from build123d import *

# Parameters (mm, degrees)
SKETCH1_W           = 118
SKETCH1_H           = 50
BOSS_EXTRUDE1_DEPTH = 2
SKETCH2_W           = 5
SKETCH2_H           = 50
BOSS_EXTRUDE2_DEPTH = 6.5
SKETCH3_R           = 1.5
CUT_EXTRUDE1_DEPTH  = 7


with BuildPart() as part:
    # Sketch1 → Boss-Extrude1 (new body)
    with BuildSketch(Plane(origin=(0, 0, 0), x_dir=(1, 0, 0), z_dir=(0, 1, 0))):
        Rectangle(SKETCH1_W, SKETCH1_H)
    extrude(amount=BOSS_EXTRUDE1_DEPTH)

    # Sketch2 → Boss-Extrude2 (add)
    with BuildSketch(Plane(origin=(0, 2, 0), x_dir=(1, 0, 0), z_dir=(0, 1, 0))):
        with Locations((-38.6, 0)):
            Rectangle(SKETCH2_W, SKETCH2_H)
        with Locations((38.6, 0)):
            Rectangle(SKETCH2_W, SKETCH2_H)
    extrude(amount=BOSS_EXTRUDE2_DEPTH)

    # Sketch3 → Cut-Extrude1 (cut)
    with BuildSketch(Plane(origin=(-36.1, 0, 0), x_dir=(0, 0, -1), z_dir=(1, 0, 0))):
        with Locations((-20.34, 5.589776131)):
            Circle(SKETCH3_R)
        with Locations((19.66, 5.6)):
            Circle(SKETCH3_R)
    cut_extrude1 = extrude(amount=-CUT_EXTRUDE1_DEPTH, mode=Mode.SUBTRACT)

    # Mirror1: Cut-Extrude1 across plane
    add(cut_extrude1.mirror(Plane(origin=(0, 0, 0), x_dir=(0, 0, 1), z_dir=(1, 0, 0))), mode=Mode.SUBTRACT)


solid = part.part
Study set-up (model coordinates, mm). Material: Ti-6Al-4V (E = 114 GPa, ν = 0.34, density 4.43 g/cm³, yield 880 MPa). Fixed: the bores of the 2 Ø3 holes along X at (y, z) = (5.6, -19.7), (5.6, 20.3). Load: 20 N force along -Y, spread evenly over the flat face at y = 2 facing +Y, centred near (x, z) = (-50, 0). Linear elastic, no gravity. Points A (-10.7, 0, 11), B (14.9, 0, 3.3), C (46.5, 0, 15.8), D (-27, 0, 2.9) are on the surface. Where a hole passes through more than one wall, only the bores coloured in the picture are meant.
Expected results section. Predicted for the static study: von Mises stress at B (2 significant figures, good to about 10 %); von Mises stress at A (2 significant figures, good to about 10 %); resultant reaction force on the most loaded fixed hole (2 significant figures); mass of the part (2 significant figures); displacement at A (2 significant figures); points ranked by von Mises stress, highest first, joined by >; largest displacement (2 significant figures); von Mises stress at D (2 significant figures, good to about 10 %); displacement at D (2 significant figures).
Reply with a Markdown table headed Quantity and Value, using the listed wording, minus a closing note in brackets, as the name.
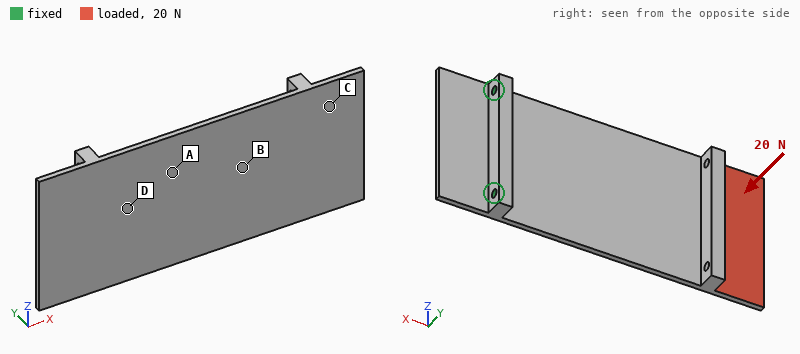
| Quantity | Value |
|---|---|
| von Mises stress at B | 35 MPa |
| von Mises stress at A | 22 MPa |
| resultant reaction force on the most loaded fixed hole | 28 N |
| mass of the part | 66 g |
| displacement at A | 0.42 mm |
| points ranked by von Mises stress, highest first, joined by > | B > A > D > C |
| largest displacement | 1.3 mm |
| von Mises stress at D | 13 MPa |
| displacement at D | 0.69 mm |
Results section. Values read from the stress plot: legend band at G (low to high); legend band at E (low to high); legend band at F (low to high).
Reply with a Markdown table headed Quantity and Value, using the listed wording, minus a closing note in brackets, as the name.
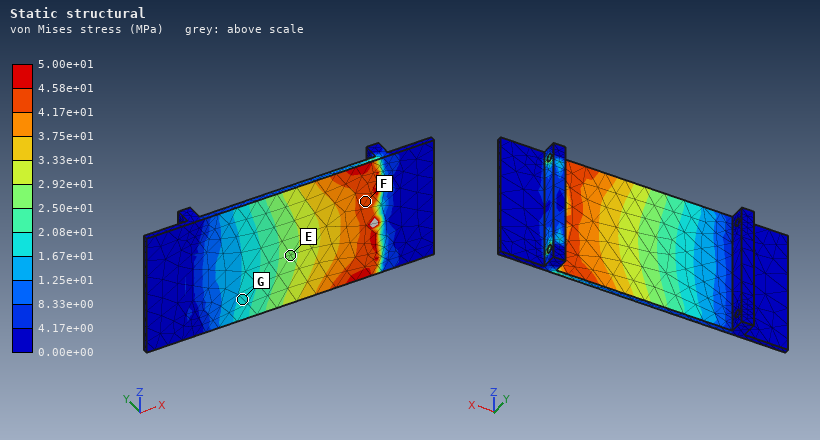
| Quantity | Value |
|---|---|
| legend band at G | 1.67e+01 to 2.08e+01 MPa |
| legend band at E | 2.50e+01 to 2.92e+01 MPa |
| legend band at F | 4.17e+01 to 4.58e+01 MPa |
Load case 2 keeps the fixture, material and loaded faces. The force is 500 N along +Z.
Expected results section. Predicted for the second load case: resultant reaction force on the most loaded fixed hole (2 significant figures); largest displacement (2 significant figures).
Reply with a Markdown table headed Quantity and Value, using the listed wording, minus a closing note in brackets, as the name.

| Quantity | Value |
|---|---|
| resultant reaction force on the most loaded fixed hole | 1.1 kN |
| largest displacement | 0.18 mm |
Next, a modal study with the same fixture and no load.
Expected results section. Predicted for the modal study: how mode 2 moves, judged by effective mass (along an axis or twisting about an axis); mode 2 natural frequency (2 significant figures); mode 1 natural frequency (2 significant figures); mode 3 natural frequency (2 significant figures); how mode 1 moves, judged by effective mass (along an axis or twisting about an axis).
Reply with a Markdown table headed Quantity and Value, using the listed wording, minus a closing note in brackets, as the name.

| Quantity | Value |
|---|---|
| how mode 2 moves, judged by effective mass | twisting about X |
| mode 2 natural frequency | 670 Hz |
| mode 1 natural frequency | 160 Hz |
| mode 3 natural frequency | 1100 Hz |
| how mode 1 moves, judged by effective mass | along Y |
